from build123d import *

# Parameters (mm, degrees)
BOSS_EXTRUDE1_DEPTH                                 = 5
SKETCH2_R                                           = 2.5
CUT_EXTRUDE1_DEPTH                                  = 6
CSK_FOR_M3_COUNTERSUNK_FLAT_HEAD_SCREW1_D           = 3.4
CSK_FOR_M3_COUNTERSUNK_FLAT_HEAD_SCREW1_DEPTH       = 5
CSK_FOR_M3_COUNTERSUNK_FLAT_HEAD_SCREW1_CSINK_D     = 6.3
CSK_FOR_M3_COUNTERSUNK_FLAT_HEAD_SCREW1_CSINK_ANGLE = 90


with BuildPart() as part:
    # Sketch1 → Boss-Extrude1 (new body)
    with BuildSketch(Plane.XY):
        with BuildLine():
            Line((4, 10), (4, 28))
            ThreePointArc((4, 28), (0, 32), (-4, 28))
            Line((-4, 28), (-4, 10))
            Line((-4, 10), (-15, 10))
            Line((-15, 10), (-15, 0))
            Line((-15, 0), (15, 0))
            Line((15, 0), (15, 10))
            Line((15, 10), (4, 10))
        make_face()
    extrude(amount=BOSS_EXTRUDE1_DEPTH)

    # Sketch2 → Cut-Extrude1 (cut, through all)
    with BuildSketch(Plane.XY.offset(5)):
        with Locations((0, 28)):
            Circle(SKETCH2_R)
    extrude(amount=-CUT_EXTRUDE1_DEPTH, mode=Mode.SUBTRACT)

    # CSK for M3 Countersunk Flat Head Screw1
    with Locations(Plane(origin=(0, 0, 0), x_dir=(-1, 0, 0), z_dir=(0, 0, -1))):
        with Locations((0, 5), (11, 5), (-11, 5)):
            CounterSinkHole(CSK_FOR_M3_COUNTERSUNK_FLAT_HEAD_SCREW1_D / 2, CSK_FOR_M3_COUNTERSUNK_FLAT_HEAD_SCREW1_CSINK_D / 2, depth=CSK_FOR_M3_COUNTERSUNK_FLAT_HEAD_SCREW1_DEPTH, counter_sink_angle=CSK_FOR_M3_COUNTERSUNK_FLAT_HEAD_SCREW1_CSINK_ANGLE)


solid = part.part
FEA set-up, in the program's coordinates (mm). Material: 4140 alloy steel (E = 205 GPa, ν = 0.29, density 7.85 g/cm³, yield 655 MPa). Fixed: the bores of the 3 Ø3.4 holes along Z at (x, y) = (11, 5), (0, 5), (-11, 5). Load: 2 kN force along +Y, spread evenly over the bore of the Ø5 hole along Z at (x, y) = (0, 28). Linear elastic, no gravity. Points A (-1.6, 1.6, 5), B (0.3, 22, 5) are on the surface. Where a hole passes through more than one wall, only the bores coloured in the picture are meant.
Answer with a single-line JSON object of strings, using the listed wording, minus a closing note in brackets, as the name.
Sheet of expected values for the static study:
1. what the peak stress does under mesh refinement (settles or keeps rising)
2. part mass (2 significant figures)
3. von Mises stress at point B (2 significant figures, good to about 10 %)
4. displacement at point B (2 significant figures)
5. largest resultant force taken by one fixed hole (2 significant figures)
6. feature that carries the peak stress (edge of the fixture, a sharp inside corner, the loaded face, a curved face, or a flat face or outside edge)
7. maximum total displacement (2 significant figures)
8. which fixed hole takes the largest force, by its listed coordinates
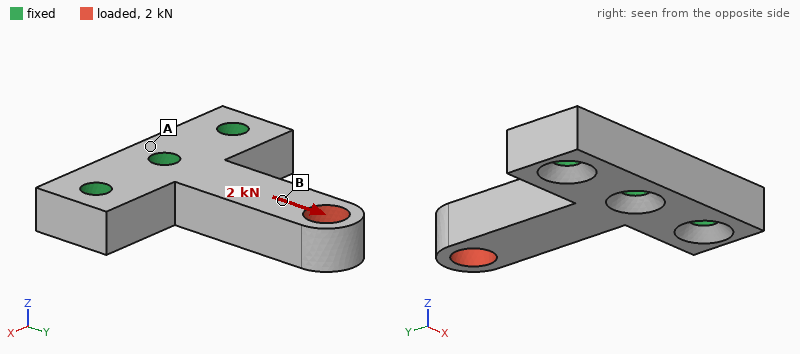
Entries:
{"what the peak stress does under mesh refinement": "keeps rising", "part mass": "16 g", "von Mises stress at point B": "32 MPa", "displacement at point B": "4.1 µm", "largest resultant force taken by one fixed hole": "1.6 kN", "feature that carries the peak stress": "edge of the fixture", "maximum total displacement": "11 µm", "which fixed hole takes the largest force, by its listed coordinates": "(0, 5)"}
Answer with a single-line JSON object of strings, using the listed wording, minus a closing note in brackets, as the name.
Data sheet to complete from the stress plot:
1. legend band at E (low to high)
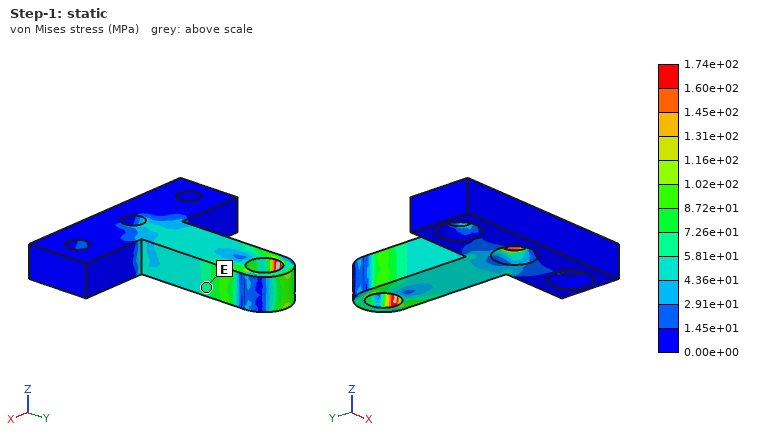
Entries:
{"legend band at E": "5.81e+01 to 7.26e+01 MPa"}
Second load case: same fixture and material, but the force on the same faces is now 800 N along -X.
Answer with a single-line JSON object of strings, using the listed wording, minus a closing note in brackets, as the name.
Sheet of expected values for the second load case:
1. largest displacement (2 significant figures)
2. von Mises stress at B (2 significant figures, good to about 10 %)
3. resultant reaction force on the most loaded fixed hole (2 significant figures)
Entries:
{"largest displacement": "83 µm", "von Mises stress at B": "66 MPa", "resultant reaction force on the most loaded fixed hole": "930 N"}
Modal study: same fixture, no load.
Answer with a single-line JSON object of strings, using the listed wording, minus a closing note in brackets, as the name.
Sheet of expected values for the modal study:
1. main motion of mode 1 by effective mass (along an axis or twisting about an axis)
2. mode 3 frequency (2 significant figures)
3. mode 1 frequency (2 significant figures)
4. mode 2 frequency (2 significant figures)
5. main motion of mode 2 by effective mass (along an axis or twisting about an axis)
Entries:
{"main motion of mode 1 by effective mass": "along Z", "mode 3 frequency": "30 kHz", "mode 1 frequency": "7200 Hz", "mode 2 frequency": "12 kHz", "main motion of mode 2 by effective mass": "along X"}
